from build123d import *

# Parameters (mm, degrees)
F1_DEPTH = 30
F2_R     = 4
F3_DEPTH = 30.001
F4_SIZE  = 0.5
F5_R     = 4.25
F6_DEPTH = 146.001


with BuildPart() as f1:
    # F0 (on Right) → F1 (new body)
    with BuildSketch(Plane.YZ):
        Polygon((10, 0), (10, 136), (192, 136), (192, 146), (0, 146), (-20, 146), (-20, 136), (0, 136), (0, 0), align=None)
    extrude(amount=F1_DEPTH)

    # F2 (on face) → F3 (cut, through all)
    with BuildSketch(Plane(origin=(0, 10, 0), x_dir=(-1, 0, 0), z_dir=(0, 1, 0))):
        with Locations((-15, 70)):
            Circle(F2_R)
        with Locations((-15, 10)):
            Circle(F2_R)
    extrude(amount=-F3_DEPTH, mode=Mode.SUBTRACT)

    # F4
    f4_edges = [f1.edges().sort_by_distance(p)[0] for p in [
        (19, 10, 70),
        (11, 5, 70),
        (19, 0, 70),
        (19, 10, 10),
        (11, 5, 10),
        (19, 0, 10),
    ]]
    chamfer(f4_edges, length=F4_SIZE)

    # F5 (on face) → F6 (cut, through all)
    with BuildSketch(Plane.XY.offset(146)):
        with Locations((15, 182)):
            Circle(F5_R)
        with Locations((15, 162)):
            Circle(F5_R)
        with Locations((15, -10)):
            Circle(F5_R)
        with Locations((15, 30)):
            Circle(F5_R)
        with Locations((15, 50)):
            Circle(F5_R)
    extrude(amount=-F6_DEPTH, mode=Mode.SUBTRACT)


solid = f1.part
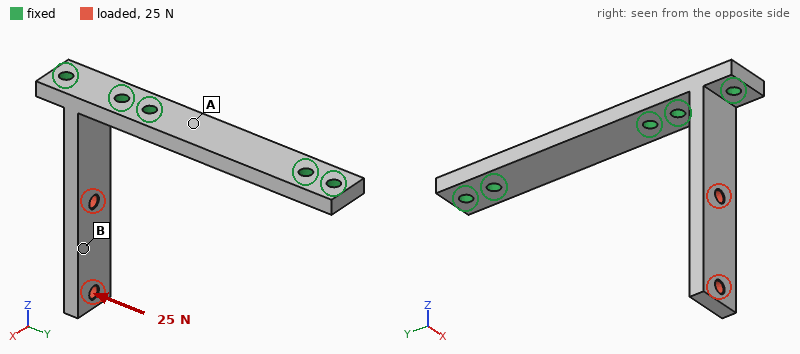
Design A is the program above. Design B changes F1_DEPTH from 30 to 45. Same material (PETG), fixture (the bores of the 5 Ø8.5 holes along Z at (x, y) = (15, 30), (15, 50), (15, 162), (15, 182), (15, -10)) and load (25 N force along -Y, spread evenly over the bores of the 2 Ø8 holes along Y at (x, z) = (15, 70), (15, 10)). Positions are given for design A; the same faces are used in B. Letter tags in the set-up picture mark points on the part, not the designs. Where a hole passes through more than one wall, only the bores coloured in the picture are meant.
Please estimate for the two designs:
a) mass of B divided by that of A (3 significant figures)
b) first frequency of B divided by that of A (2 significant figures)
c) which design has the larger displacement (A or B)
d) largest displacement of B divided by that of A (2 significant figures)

1.52
0.99
A
0.68
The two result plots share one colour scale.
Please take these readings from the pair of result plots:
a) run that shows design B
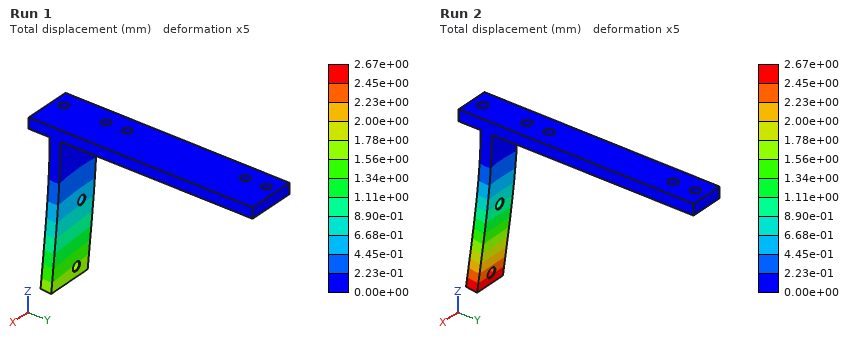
Run 1
